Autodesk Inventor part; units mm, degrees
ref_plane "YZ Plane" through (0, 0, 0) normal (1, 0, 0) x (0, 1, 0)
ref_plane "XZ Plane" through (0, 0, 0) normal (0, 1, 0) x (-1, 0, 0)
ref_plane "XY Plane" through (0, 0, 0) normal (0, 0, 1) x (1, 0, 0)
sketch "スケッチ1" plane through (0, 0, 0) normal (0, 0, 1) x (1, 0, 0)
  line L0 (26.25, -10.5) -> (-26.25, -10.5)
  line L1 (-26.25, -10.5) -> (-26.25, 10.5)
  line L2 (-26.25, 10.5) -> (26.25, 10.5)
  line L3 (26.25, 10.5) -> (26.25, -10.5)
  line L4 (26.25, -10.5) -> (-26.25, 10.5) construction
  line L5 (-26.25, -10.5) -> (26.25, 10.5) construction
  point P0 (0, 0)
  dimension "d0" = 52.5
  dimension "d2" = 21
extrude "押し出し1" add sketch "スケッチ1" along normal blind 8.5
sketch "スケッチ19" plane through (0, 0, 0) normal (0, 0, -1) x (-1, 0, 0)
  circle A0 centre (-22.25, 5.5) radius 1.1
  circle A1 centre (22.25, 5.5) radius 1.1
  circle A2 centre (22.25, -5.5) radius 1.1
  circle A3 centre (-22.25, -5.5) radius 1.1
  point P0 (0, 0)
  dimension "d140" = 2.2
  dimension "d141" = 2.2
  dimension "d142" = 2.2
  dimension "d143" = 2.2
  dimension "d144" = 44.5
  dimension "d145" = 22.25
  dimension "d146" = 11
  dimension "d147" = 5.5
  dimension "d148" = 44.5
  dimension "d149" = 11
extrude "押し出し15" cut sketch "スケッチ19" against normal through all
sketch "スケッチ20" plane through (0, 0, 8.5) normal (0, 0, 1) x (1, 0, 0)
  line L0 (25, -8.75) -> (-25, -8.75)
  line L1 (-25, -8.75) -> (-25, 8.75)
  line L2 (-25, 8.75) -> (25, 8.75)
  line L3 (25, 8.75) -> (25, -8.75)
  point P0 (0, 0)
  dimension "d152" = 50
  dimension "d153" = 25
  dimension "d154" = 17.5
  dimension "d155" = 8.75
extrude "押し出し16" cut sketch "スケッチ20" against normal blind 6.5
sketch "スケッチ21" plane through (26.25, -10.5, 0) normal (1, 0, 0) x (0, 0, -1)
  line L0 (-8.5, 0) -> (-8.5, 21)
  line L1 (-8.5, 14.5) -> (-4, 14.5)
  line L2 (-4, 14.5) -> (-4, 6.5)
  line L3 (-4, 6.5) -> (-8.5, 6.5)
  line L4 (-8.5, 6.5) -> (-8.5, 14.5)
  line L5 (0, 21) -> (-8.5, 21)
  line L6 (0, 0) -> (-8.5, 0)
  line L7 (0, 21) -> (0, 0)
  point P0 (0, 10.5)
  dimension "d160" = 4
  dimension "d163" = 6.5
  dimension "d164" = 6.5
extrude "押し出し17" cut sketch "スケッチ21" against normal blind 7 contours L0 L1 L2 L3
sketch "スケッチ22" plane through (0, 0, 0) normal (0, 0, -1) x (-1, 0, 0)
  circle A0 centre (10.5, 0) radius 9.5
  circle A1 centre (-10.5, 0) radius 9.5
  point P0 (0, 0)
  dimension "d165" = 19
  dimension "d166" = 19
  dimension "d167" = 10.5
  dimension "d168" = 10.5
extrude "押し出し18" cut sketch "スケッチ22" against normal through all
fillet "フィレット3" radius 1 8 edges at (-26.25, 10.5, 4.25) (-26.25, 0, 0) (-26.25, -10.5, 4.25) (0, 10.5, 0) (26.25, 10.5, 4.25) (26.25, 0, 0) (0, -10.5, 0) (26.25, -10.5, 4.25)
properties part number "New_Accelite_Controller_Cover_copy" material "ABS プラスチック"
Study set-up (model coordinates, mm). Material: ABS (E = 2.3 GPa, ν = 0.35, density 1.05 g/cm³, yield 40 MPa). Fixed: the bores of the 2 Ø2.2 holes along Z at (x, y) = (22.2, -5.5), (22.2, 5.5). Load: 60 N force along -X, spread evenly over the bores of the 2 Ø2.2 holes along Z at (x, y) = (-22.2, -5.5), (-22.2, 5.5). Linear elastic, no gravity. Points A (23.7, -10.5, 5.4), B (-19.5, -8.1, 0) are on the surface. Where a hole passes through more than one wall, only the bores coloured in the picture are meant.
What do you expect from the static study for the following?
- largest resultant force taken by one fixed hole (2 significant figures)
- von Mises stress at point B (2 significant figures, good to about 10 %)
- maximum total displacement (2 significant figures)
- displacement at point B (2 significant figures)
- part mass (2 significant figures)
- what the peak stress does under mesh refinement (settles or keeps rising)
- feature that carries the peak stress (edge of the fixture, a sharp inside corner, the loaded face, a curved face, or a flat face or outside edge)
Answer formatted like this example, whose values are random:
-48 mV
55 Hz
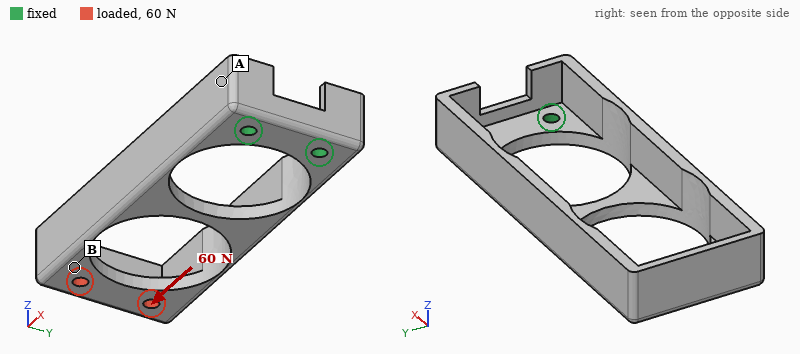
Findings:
30 N
4.0 MPa
0.67 mm
0.52 mm
2.5 g
keeps rising
a sharp inside corner
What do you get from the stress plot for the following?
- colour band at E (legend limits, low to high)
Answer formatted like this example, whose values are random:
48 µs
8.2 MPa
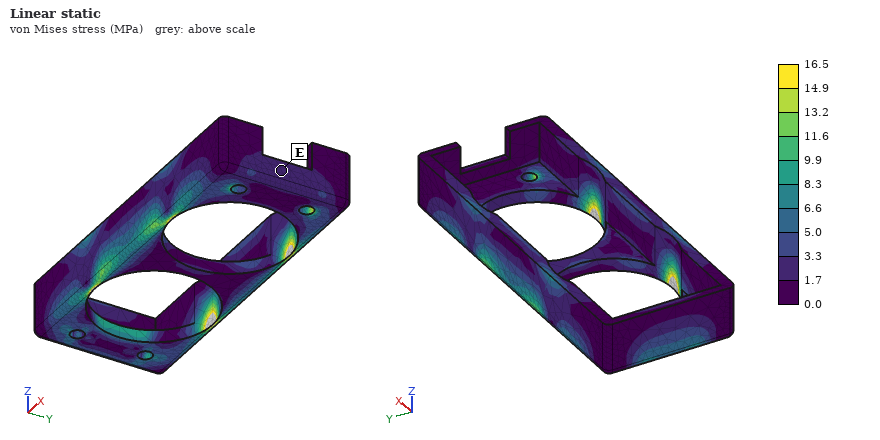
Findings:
1.7 to 3.3 MPa
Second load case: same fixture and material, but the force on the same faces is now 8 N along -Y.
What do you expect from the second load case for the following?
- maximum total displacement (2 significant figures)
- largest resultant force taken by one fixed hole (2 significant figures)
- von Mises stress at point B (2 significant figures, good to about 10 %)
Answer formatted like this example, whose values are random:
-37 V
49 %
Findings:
0.63 mm
23 N
1.9 MPa
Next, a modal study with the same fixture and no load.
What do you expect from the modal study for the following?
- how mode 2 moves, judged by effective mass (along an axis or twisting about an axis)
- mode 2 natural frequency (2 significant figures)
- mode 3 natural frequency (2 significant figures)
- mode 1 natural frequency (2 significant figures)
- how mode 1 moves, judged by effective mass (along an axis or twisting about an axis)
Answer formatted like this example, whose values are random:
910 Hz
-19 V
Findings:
along Y
520 Hz
700 Hz
350 Hz
along Z
